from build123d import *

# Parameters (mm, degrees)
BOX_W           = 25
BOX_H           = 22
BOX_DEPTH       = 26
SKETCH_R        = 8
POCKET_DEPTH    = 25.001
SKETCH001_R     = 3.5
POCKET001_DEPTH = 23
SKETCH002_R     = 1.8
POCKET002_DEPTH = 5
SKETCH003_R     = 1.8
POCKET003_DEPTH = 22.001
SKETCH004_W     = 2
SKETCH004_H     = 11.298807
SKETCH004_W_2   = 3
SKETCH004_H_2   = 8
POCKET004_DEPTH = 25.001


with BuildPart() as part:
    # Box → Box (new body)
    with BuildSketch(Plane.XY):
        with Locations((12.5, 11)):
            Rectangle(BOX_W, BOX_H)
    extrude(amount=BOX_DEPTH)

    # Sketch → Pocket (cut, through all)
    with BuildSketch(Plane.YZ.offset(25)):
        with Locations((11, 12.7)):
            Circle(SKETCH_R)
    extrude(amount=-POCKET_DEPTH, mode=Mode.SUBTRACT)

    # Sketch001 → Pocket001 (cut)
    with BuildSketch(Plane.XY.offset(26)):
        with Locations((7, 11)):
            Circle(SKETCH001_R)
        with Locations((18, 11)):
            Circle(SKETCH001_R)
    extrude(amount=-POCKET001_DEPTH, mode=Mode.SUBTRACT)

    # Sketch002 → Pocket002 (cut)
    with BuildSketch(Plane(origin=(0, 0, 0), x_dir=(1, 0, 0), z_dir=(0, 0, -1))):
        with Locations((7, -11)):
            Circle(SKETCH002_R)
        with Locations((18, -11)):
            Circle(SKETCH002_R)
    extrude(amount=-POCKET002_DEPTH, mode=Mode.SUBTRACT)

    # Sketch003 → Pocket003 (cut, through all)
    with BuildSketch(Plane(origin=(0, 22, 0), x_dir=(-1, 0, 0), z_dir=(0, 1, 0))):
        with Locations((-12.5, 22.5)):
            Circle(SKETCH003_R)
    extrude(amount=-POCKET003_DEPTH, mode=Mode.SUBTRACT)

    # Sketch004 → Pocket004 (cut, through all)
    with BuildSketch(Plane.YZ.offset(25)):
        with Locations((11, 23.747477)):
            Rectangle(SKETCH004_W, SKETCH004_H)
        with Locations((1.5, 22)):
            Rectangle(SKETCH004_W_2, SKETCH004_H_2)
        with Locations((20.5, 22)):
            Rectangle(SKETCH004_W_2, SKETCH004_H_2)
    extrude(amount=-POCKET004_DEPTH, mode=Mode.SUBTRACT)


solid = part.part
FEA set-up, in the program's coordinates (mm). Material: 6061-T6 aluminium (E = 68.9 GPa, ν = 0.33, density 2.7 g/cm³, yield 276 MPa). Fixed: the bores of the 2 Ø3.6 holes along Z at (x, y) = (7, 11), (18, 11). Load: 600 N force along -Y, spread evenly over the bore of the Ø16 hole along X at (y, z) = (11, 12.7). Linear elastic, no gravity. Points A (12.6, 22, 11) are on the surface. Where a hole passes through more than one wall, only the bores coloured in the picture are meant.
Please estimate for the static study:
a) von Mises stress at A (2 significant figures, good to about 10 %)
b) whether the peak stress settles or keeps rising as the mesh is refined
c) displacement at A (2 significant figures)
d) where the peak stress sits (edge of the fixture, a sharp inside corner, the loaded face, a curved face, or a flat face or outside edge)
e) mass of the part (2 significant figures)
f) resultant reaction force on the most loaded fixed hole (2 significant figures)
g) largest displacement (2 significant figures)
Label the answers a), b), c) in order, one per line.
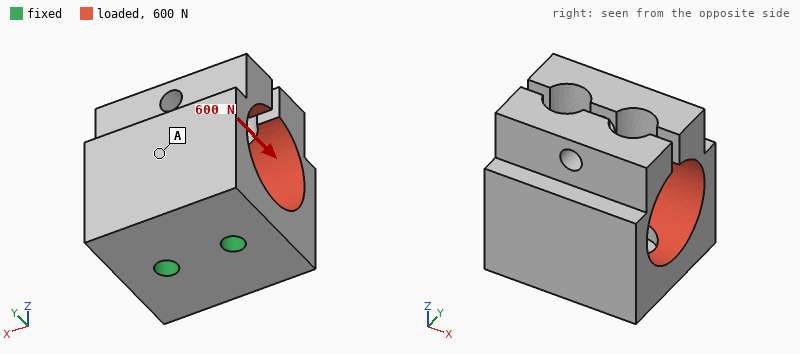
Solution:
a) 19 MPa
b) keeps rising
c) 35 µm
d) edge of the fixture
e) 19 g
f) 300 N
g) 87 µm
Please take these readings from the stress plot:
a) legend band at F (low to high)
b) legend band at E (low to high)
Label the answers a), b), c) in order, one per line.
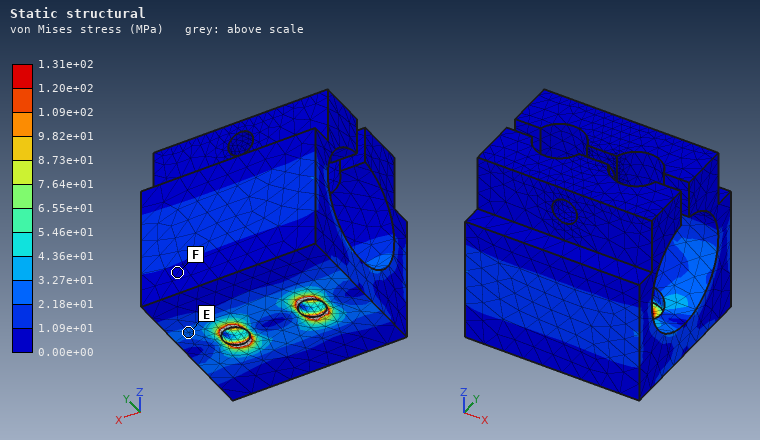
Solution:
a) 0.00e+00 to 1.09e+01 MPa
b) 2.18e+01 to 3.27e+01 MPa
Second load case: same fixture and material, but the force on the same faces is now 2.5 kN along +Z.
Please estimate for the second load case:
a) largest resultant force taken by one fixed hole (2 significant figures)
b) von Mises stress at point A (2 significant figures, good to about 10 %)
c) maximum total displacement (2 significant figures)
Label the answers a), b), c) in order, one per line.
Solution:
a) 1.3 kN
b) 41 MPa
c) 69 µm
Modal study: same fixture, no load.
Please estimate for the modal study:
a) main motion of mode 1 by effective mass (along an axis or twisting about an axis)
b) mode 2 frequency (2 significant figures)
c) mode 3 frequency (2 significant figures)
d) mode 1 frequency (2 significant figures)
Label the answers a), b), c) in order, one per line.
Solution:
a) along Y
b) 4200 Hz
c) 7100 Hz
d) 3500 Hz
